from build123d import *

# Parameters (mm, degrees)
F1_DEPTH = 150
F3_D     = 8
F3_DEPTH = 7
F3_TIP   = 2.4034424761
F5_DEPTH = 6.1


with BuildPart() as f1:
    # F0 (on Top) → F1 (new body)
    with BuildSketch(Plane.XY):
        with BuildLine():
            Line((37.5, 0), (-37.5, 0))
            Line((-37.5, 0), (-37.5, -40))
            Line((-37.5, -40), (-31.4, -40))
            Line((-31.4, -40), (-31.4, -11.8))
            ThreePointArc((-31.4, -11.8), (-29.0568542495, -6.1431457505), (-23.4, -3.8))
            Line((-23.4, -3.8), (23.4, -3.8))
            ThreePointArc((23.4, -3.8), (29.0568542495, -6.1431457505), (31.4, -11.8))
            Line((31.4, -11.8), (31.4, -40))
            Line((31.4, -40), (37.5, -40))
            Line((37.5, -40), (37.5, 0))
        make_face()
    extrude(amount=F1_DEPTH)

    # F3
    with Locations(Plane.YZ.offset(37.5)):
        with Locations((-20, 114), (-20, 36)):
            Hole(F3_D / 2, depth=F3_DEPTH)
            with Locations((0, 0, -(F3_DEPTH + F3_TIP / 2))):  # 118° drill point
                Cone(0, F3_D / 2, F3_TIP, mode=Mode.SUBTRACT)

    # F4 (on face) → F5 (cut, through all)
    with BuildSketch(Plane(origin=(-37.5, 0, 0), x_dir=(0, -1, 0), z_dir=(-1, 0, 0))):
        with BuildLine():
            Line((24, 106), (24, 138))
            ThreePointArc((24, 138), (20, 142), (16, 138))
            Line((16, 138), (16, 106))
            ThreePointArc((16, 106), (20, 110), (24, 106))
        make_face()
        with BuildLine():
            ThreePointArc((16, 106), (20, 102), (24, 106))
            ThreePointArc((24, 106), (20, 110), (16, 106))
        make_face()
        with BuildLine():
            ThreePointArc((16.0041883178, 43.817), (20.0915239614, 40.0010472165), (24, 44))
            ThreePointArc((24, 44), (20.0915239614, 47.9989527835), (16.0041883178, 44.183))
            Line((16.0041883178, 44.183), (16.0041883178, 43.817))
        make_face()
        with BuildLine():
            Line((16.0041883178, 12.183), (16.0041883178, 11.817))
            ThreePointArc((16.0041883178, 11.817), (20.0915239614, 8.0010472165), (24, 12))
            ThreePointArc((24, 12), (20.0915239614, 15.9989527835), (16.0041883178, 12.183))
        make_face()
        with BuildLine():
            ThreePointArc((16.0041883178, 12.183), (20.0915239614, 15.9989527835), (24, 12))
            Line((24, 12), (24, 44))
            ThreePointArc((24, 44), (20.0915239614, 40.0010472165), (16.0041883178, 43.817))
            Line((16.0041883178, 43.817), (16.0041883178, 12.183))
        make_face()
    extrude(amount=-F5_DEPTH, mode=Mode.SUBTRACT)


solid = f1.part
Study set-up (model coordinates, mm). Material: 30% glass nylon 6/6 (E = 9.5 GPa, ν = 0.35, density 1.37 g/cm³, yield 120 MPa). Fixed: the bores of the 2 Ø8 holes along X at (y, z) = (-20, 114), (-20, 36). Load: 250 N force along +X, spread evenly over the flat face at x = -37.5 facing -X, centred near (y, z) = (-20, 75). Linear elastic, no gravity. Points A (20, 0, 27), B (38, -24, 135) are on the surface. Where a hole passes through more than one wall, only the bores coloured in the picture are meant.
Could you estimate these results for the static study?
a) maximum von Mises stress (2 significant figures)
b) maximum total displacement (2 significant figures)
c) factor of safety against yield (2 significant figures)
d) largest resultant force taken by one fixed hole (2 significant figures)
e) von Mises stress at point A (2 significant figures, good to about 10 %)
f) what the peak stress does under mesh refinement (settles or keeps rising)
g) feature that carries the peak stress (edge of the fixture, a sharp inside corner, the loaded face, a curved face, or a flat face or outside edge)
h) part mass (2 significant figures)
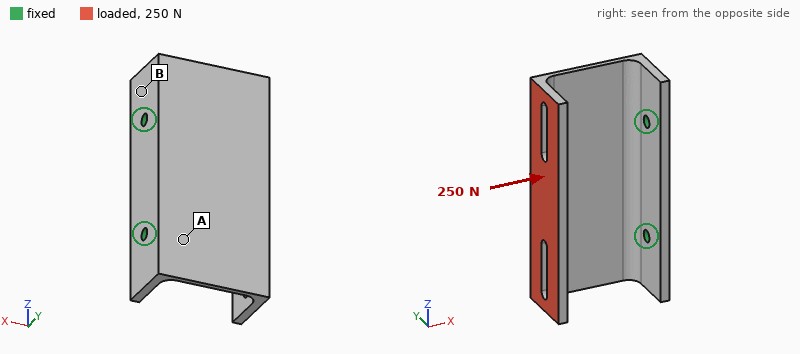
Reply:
13 MPa
2.0 mm
9.2
130 N
11 MPa
settles
a curved face
150 g
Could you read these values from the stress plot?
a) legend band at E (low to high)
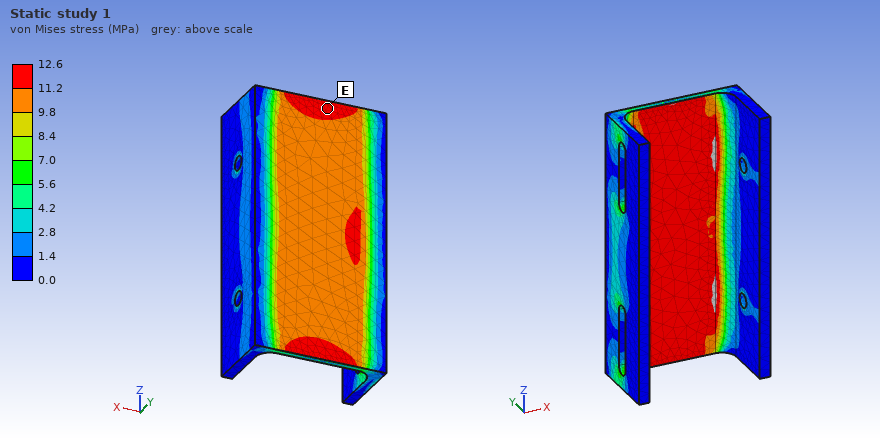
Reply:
11.2 to 12.6 MPa
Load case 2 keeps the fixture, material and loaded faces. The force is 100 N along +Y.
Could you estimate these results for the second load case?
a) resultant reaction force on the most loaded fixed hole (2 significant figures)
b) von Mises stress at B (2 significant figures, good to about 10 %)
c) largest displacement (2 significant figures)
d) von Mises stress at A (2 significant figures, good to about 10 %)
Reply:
50 N
2.9 MPa
2.1 mm
14 MPa
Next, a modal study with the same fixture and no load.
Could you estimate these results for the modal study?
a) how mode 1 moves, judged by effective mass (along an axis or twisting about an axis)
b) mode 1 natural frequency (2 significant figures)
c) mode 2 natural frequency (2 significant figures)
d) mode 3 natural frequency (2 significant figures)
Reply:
along Y
160 Hz
310 Hz
650 Hz
